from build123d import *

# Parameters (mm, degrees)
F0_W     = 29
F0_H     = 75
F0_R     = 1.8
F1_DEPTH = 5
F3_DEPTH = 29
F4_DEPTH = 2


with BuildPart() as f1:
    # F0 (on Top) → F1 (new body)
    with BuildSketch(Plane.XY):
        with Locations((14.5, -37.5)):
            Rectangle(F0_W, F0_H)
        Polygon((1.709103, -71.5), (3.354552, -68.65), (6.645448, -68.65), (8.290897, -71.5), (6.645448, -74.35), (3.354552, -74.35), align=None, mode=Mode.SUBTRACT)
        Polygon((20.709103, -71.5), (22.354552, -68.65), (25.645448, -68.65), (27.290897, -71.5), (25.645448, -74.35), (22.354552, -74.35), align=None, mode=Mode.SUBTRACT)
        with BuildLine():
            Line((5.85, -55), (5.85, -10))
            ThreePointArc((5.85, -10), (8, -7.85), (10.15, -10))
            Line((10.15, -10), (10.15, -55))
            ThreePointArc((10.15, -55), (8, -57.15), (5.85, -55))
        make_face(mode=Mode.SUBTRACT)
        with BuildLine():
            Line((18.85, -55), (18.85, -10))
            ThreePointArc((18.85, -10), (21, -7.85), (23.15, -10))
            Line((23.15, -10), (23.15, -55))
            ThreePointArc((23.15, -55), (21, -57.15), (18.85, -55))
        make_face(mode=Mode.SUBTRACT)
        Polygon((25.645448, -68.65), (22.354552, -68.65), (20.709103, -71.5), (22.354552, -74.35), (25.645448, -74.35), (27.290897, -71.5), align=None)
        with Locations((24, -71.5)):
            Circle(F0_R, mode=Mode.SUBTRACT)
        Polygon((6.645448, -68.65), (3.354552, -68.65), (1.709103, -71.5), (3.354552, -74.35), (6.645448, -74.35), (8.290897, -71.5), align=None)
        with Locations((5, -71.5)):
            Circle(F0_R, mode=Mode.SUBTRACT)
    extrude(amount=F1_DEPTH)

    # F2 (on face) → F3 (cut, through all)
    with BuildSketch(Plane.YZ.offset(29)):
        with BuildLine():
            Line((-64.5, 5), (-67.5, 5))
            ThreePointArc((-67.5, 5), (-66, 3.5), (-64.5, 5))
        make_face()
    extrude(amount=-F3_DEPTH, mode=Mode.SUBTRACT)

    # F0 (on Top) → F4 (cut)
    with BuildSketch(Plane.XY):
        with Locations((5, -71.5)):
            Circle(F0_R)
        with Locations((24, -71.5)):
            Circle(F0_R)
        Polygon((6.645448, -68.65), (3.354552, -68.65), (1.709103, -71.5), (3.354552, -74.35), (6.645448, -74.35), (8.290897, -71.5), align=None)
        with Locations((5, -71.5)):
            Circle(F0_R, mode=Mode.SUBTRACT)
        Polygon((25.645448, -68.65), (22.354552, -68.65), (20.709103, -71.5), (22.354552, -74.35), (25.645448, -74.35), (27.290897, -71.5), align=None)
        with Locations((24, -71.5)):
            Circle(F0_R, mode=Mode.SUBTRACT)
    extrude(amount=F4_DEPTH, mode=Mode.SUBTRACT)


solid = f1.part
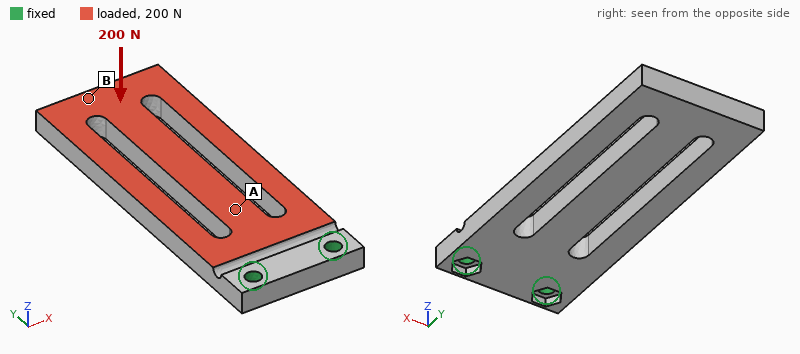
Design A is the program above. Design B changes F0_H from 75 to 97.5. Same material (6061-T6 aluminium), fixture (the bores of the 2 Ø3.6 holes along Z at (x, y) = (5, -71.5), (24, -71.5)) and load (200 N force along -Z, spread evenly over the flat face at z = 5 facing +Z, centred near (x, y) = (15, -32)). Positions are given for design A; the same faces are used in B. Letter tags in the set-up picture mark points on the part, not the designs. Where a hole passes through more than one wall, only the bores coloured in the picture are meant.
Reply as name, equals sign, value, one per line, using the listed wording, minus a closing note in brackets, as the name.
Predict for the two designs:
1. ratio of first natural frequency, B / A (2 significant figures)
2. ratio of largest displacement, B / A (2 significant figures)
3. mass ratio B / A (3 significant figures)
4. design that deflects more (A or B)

ratio of first natural frequency, B / A = 0.73
ratio of largest displacement, B / A = 1.5
mass ratio B / A = 1.38
design that deflects more = B
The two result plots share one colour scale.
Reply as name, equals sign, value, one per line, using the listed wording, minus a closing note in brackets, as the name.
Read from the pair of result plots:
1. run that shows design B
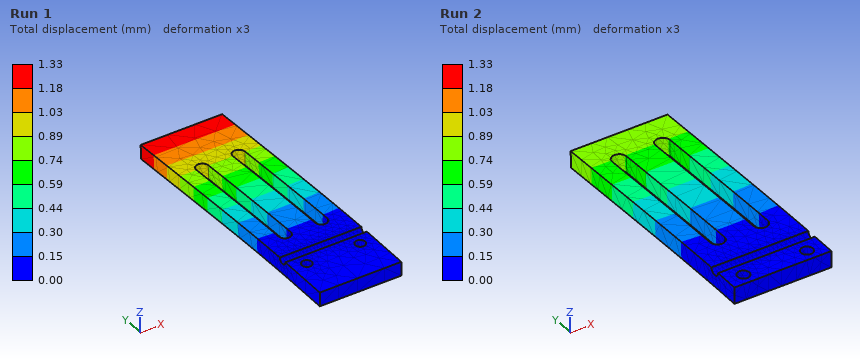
run that shows design B = Run 1
